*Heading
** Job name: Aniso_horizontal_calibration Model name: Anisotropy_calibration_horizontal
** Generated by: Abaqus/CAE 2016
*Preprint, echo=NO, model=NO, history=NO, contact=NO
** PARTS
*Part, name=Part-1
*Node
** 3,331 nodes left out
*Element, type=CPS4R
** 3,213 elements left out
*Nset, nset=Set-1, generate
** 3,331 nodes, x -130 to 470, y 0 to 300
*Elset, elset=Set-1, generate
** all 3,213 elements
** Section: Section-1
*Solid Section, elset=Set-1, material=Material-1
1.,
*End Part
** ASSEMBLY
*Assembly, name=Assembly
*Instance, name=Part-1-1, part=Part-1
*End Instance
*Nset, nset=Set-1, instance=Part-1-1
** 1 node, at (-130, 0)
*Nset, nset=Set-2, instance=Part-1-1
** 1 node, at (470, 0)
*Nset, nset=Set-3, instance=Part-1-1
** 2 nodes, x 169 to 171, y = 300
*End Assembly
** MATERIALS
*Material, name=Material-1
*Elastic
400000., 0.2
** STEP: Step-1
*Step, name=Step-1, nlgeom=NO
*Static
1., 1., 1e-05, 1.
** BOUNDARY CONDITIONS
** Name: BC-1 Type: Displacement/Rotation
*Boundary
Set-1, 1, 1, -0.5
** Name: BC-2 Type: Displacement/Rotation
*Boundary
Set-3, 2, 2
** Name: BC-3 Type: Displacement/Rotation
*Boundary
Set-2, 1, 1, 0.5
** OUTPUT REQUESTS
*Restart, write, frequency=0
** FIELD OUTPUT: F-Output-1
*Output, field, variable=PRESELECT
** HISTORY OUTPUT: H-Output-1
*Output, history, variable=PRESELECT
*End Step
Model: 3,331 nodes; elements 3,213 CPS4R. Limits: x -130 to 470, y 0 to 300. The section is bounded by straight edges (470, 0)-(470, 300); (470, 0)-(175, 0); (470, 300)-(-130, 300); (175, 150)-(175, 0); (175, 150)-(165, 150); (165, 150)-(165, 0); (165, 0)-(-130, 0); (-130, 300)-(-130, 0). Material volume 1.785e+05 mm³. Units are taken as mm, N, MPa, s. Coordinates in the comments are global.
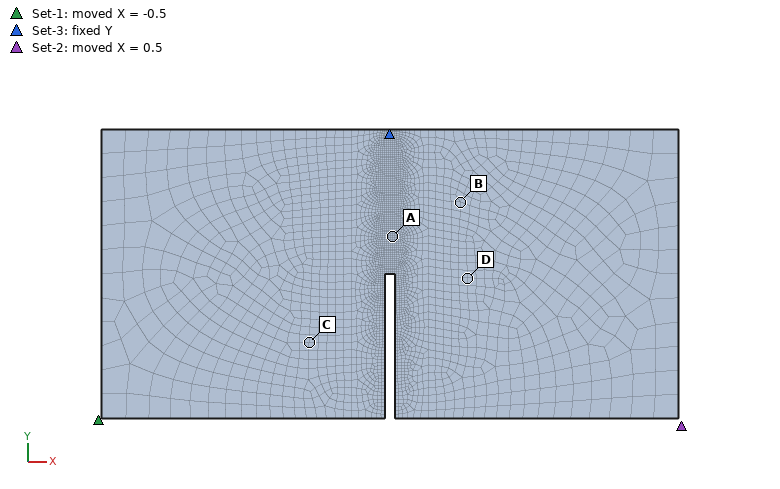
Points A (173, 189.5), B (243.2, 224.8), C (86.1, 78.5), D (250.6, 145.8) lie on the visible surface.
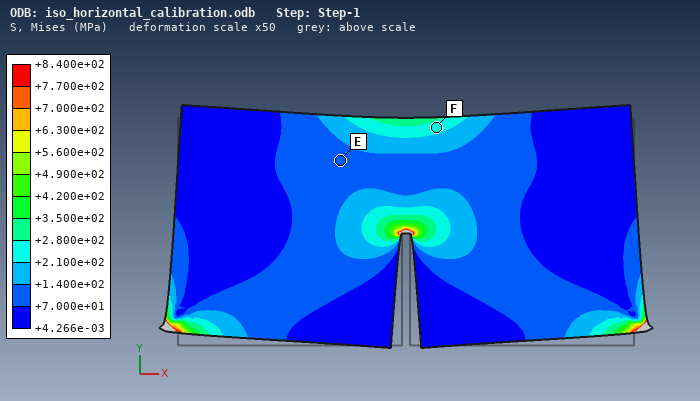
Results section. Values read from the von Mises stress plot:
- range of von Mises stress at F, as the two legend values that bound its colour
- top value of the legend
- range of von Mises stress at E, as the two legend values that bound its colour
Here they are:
+2.100e+02 to +2.800e+02 MPa
+8.400e+02 MPa
+7.000e+01 to +1.400e+02 MPa
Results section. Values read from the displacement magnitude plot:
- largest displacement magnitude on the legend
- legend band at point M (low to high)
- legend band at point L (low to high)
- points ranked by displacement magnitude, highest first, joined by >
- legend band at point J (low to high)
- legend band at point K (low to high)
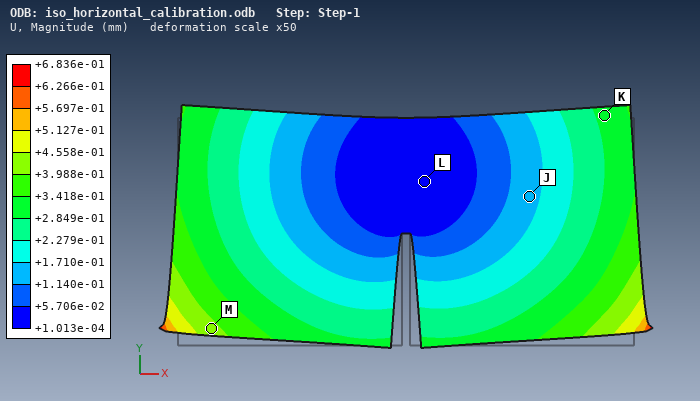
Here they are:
+6.836e-01 mm
+3.988e-01 to +4.558e-01 mm
+1.013e-04 to +5.706e-02 mm
M > K > J > L
+1.140e-01 to +1.710e-01 mm
+2.849e-01 to +3.418e-01 mm
